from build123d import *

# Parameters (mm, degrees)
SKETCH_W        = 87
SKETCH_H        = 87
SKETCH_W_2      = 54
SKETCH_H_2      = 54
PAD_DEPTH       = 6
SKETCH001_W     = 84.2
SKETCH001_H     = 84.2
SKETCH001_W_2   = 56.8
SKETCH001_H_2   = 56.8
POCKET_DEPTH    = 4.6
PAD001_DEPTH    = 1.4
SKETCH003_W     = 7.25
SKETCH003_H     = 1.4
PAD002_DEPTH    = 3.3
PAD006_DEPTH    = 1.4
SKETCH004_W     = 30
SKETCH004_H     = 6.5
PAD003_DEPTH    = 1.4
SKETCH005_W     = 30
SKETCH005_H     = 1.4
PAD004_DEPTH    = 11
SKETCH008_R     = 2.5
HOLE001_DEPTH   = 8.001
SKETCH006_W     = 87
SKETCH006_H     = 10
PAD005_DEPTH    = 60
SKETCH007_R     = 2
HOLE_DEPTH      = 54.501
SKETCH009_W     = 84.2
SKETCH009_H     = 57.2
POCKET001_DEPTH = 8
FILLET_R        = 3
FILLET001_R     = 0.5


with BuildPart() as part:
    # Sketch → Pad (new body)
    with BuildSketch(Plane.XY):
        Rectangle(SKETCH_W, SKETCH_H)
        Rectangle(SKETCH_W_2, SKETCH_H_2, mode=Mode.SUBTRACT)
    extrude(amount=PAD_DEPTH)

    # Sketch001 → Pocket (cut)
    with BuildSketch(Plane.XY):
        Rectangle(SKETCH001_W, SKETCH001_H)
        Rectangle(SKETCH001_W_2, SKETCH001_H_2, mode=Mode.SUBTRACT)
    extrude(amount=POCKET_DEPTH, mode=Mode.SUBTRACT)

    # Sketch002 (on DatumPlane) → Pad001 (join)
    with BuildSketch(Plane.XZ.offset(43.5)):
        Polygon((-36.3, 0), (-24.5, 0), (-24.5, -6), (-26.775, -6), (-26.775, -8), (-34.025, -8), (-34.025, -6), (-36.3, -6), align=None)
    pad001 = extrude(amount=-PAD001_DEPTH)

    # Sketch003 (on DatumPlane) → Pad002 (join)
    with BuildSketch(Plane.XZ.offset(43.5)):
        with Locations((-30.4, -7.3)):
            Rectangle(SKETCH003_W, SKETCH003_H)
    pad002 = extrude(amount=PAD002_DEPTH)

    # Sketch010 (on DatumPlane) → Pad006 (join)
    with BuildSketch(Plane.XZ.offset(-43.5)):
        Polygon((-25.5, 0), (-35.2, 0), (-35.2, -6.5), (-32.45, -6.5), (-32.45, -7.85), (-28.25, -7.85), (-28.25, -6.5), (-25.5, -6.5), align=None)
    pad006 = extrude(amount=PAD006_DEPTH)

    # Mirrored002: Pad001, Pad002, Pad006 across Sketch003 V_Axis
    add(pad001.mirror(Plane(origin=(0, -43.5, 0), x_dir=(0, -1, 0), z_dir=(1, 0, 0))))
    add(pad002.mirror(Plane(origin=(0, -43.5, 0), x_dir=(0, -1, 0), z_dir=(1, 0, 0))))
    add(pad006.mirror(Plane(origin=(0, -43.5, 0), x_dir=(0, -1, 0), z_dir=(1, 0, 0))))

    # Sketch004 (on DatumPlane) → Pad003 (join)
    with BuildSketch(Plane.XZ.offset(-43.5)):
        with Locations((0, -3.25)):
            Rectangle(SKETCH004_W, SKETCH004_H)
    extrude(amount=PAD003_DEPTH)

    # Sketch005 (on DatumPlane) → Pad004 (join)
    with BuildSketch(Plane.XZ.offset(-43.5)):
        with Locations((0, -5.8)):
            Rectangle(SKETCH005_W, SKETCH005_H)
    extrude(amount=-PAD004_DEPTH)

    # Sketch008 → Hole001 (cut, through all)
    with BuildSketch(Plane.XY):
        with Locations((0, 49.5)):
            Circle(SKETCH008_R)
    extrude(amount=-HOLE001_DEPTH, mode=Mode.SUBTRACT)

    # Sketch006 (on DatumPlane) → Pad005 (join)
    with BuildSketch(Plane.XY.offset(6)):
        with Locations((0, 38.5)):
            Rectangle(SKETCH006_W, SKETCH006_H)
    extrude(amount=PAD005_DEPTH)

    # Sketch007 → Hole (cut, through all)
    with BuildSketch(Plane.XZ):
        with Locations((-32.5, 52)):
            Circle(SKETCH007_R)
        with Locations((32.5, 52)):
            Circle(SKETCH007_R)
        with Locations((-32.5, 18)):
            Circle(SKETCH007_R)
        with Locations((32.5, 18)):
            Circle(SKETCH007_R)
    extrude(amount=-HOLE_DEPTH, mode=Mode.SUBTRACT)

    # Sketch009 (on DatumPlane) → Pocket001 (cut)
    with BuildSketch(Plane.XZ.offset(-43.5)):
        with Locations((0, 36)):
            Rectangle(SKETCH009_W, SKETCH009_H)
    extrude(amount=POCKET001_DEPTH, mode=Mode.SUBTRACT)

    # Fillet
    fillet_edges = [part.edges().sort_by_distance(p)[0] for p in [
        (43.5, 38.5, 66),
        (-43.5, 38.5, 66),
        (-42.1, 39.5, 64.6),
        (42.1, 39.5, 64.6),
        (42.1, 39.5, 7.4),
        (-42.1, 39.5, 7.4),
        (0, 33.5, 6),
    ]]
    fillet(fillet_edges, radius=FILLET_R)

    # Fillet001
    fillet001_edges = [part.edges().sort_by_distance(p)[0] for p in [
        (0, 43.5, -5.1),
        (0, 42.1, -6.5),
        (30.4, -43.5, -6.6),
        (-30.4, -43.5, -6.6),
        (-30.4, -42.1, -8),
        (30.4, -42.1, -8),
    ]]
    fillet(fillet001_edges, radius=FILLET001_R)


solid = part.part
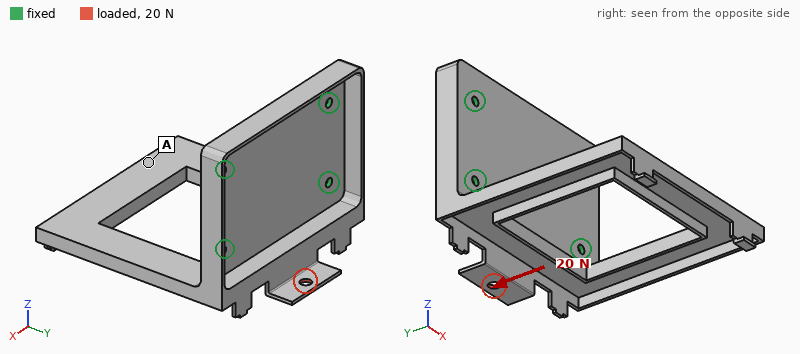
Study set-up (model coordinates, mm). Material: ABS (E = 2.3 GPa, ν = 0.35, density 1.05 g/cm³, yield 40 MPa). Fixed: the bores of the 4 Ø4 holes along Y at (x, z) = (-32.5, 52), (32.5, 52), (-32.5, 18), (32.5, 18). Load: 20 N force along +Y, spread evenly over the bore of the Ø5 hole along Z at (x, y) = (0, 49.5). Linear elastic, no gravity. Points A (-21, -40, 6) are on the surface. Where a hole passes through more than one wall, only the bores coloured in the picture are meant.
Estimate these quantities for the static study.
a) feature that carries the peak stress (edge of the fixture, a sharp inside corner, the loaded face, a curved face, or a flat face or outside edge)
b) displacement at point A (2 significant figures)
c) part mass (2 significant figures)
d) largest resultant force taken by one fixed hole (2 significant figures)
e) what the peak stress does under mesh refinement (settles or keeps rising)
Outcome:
a sharp inside corner
0.51 mm
26 g
17 N
keeps rising
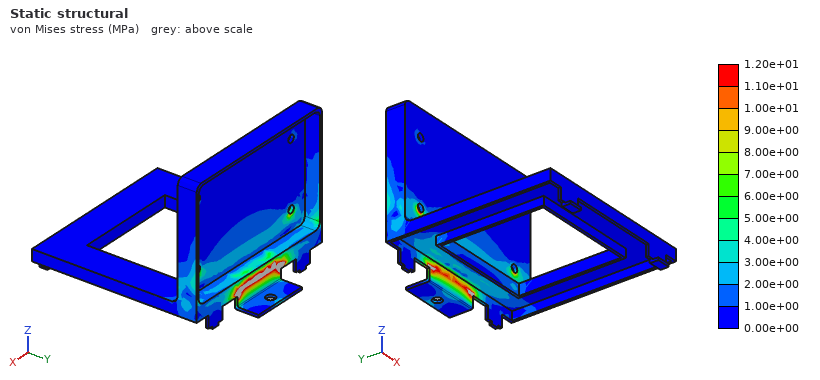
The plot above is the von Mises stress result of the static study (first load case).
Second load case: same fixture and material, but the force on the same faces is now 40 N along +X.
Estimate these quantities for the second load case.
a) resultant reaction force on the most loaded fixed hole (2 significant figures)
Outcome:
25 N
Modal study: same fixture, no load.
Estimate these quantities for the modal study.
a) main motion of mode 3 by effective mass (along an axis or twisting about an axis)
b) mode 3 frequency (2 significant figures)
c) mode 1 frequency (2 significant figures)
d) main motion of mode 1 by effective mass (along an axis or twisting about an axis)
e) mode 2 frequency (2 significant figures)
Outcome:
along X
430 Hz
100 Hz
along Z
170 Hz
